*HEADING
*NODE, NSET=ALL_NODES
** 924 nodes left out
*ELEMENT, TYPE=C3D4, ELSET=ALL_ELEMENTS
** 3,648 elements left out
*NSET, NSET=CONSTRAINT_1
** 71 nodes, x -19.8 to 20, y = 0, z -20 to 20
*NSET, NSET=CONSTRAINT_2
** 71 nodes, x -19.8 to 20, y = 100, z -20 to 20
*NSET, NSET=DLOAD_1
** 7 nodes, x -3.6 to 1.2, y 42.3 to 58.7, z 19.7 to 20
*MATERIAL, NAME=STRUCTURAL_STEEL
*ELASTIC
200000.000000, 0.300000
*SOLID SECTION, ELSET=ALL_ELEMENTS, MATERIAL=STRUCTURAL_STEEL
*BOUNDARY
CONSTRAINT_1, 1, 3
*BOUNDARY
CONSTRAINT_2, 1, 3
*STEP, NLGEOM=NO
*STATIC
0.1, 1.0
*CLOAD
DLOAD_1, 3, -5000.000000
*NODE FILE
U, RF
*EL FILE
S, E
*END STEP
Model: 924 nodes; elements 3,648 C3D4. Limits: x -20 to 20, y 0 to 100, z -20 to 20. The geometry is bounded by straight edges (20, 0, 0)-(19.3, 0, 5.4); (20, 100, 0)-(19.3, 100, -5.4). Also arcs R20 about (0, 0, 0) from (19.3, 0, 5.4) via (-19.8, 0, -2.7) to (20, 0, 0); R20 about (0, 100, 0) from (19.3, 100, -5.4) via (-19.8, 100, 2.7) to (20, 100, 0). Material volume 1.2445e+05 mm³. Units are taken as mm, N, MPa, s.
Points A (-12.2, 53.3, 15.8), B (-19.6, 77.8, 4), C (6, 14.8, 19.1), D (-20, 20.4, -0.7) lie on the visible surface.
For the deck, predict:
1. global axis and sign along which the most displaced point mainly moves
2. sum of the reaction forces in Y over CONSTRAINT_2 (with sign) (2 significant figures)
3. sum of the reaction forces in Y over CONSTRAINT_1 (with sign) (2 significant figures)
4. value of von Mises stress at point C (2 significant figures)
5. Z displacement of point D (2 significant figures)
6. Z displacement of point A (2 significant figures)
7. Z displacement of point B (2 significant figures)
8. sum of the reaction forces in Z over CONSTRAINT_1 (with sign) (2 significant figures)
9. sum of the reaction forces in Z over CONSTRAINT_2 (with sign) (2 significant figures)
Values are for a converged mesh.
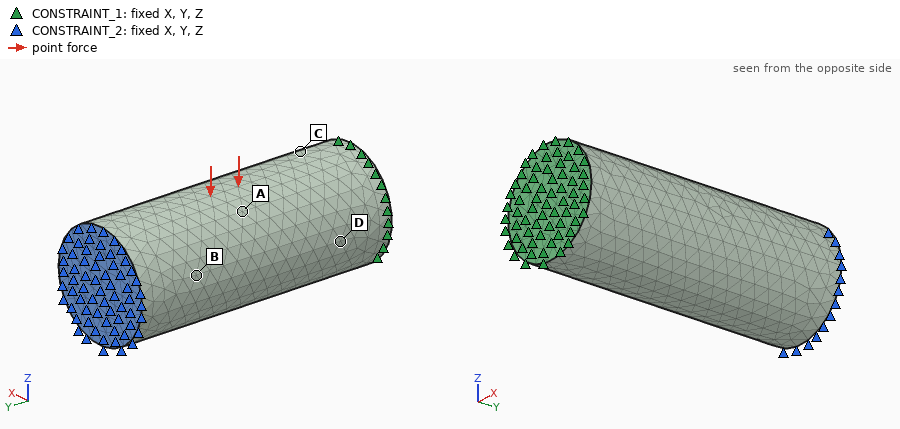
-Z
-2100 N
2100 N
24 MPa
-0.0069 mm
-0.016 mm
-0.0078 mm
17000 N
18000 N
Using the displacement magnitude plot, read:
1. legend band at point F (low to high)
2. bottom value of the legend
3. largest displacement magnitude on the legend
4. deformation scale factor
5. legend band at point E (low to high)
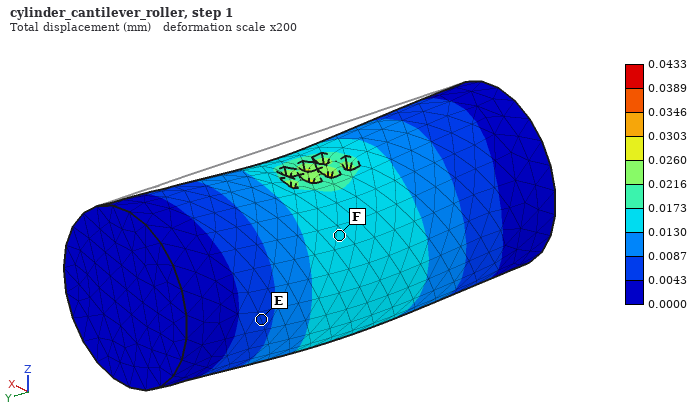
0.0130 to 0.0173 mm
0.0000 mm
0.0433 mm
200
0.0043 to 0.0087 mm
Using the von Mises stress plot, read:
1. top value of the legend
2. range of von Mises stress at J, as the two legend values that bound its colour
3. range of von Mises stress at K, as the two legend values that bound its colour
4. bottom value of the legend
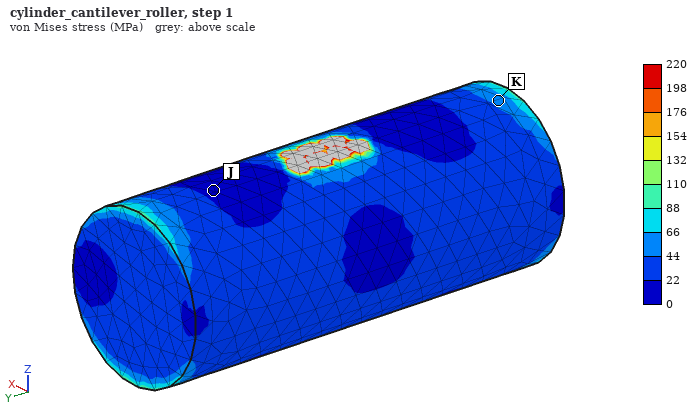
220 MPa
0 to 22 MPa
44 to 66 MPa
0 MPa
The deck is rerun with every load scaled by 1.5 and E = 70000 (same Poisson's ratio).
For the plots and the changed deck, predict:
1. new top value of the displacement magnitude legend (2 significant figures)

0.19 mm
